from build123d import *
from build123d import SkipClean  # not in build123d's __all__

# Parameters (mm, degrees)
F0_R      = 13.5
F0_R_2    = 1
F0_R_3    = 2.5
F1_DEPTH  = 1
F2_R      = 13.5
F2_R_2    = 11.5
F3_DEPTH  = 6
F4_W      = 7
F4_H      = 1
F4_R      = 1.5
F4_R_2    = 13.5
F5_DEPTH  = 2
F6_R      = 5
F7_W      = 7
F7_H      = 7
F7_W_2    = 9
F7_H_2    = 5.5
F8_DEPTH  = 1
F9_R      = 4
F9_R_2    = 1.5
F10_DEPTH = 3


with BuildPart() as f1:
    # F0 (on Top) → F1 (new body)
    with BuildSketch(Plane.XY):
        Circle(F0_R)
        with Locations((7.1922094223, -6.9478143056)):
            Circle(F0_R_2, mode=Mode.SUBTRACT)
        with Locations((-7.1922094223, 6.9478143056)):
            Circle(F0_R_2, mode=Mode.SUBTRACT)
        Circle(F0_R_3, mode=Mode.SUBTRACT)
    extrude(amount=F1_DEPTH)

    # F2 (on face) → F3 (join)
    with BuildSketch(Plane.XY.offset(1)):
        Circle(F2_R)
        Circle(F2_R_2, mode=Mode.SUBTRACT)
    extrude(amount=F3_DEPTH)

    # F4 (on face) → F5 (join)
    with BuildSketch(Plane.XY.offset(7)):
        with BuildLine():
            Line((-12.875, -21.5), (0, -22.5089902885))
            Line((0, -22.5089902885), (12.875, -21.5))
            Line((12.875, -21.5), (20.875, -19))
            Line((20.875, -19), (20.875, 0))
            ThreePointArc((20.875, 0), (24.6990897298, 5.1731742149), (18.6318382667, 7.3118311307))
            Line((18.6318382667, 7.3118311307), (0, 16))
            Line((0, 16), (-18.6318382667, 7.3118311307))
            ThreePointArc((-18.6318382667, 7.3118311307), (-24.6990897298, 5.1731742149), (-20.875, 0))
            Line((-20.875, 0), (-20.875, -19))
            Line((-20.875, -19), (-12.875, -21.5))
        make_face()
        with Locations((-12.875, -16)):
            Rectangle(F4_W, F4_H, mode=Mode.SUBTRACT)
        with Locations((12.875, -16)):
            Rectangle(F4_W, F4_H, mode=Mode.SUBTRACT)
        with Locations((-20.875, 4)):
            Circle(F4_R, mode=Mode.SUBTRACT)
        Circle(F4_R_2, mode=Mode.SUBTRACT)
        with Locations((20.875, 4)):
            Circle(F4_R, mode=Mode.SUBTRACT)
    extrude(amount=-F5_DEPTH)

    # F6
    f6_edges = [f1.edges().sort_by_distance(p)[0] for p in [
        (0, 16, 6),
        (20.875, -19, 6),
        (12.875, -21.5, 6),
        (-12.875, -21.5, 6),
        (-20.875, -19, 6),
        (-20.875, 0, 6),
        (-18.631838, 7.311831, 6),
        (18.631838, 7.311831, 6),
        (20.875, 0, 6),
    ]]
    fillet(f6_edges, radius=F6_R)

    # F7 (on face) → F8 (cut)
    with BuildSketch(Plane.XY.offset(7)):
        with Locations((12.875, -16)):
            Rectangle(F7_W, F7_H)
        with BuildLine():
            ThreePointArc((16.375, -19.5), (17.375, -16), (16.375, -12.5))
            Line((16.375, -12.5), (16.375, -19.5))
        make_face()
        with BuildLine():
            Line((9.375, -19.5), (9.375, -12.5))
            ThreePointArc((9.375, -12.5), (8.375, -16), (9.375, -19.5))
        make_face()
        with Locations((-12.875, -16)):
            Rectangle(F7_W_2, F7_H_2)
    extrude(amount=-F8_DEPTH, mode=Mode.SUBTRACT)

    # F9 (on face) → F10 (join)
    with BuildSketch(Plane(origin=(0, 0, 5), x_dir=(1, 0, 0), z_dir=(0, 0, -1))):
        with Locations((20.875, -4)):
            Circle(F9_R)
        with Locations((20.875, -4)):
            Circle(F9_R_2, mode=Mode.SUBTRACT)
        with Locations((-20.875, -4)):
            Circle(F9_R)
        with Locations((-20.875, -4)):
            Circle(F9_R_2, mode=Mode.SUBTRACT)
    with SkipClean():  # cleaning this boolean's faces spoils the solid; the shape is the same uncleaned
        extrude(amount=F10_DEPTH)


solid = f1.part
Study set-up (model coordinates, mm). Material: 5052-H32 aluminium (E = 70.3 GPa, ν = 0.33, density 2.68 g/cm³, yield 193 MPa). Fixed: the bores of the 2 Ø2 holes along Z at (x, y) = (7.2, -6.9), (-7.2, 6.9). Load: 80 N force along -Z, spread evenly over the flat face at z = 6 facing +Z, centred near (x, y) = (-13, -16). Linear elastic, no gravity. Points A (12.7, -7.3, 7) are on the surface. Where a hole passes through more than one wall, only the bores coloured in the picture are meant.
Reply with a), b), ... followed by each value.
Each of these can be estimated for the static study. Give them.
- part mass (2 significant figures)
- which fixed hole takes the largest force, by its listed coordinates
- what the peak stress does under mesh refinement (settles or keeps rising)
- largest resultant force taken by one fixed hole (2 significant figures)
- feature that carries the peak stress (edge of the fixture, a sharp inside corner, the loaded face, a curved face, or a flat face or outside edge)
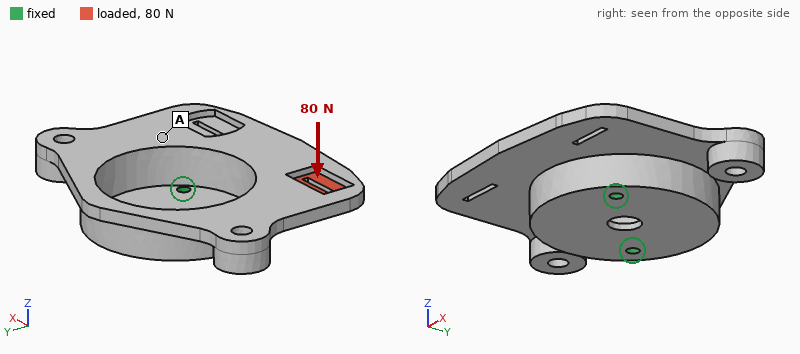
a) 8.8 g
b) (7.2, -6.9)
c) keeps rising
d) 47 N
e) edge of the fixture
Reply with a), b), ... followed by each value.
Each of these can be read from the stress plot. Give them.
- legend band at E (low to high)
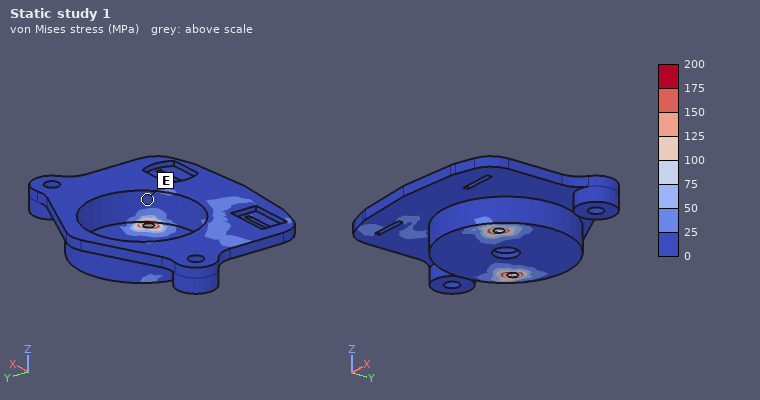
a) 0 to 25 MPa
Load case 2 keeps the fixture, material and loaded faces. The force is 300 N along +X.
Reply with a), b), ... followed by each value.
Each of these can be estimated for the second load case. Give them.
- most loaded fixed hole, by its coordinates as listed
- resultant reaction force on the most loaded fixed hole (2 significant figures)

a) (7.2, -6.9)
b) 360 N
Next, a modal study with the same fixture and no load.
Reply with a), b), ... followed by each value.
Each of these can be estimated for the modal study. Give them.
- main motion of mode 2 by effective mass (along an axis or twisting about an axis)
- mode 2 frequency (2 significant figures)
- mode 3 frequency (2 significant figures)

a) along Z
b) 6500 Hz
c) 7300 Hz
